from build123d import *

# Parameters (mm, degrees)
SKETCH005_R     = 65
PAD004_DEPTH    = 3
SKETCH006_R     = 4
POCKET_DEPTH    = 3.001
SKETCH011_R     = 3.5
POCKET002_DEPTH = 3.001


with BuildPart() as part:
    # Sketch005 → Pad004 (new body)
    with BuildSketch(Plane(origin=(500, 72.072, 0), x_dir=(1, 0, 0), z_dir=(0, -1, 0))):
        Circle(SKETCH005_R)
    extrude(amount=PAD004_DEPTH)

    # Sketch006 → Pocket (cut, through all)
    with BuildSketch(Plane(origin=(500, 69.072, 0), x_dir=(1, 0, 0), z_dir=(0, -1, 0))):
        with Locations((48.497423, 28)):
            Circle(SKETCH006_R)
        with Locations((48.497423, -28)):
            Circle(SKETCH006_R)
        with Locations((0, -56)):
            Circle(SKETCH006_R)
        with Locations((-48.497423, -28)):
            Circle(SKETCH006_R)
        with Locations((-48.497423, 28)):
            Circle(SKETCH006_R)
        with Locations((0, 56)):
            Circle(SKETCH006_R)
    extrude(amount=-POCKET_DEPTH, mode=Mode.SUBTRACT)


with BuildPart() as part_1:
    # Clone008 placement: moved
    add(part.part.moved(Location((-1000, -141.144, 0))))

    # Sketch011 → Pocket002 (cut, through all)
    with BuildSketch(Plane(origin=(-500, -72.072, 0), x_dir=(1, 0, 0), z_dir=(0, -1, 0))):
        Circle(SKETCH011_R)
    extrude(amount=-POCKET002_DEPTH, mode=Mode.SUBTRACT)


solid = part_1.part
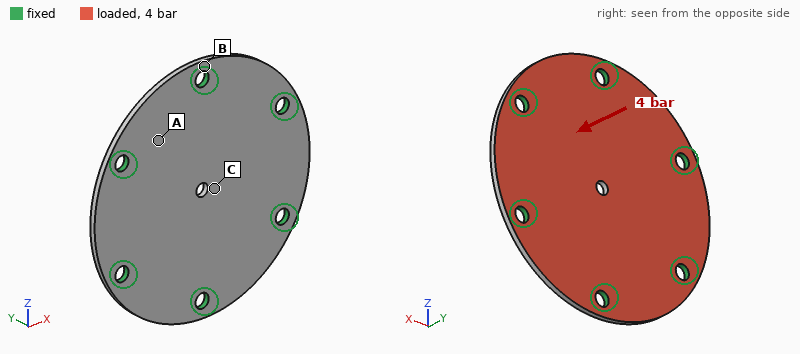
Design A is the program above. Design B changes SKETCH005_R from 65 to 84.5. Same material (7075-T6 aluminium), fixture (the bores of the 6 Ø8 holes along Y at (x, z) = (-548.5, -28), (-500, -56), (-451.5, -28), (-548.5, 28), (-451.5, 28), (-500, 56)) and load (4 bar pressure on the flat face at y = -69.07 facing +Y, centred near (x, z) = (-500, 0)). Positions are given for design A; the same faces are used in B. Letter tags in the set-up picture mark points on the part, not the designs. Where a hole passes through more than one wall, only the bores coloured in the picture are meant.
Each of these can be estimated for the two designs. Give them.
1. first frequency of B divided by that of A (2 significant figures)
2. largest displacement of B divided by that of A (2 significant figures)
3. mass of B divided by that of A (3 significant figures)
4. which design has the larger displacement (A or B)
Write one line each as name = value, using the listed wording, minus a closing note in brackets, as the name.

first frequency of B divided by that of A = 0.96
largest displacement of B divided by that of A = 0.84
mass of B divided by that of A = 1.71
which design has the larger displacement = A
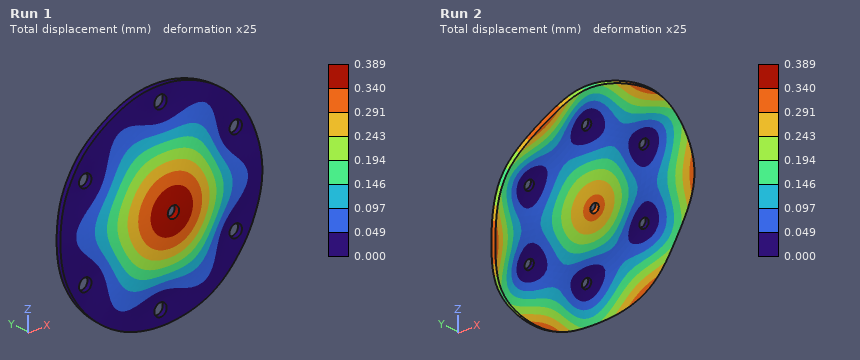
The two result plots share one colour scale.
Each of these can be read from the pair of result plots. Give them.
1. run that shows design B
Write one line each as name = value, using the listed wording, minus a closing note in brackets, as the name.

run that shows design B = Run 2
